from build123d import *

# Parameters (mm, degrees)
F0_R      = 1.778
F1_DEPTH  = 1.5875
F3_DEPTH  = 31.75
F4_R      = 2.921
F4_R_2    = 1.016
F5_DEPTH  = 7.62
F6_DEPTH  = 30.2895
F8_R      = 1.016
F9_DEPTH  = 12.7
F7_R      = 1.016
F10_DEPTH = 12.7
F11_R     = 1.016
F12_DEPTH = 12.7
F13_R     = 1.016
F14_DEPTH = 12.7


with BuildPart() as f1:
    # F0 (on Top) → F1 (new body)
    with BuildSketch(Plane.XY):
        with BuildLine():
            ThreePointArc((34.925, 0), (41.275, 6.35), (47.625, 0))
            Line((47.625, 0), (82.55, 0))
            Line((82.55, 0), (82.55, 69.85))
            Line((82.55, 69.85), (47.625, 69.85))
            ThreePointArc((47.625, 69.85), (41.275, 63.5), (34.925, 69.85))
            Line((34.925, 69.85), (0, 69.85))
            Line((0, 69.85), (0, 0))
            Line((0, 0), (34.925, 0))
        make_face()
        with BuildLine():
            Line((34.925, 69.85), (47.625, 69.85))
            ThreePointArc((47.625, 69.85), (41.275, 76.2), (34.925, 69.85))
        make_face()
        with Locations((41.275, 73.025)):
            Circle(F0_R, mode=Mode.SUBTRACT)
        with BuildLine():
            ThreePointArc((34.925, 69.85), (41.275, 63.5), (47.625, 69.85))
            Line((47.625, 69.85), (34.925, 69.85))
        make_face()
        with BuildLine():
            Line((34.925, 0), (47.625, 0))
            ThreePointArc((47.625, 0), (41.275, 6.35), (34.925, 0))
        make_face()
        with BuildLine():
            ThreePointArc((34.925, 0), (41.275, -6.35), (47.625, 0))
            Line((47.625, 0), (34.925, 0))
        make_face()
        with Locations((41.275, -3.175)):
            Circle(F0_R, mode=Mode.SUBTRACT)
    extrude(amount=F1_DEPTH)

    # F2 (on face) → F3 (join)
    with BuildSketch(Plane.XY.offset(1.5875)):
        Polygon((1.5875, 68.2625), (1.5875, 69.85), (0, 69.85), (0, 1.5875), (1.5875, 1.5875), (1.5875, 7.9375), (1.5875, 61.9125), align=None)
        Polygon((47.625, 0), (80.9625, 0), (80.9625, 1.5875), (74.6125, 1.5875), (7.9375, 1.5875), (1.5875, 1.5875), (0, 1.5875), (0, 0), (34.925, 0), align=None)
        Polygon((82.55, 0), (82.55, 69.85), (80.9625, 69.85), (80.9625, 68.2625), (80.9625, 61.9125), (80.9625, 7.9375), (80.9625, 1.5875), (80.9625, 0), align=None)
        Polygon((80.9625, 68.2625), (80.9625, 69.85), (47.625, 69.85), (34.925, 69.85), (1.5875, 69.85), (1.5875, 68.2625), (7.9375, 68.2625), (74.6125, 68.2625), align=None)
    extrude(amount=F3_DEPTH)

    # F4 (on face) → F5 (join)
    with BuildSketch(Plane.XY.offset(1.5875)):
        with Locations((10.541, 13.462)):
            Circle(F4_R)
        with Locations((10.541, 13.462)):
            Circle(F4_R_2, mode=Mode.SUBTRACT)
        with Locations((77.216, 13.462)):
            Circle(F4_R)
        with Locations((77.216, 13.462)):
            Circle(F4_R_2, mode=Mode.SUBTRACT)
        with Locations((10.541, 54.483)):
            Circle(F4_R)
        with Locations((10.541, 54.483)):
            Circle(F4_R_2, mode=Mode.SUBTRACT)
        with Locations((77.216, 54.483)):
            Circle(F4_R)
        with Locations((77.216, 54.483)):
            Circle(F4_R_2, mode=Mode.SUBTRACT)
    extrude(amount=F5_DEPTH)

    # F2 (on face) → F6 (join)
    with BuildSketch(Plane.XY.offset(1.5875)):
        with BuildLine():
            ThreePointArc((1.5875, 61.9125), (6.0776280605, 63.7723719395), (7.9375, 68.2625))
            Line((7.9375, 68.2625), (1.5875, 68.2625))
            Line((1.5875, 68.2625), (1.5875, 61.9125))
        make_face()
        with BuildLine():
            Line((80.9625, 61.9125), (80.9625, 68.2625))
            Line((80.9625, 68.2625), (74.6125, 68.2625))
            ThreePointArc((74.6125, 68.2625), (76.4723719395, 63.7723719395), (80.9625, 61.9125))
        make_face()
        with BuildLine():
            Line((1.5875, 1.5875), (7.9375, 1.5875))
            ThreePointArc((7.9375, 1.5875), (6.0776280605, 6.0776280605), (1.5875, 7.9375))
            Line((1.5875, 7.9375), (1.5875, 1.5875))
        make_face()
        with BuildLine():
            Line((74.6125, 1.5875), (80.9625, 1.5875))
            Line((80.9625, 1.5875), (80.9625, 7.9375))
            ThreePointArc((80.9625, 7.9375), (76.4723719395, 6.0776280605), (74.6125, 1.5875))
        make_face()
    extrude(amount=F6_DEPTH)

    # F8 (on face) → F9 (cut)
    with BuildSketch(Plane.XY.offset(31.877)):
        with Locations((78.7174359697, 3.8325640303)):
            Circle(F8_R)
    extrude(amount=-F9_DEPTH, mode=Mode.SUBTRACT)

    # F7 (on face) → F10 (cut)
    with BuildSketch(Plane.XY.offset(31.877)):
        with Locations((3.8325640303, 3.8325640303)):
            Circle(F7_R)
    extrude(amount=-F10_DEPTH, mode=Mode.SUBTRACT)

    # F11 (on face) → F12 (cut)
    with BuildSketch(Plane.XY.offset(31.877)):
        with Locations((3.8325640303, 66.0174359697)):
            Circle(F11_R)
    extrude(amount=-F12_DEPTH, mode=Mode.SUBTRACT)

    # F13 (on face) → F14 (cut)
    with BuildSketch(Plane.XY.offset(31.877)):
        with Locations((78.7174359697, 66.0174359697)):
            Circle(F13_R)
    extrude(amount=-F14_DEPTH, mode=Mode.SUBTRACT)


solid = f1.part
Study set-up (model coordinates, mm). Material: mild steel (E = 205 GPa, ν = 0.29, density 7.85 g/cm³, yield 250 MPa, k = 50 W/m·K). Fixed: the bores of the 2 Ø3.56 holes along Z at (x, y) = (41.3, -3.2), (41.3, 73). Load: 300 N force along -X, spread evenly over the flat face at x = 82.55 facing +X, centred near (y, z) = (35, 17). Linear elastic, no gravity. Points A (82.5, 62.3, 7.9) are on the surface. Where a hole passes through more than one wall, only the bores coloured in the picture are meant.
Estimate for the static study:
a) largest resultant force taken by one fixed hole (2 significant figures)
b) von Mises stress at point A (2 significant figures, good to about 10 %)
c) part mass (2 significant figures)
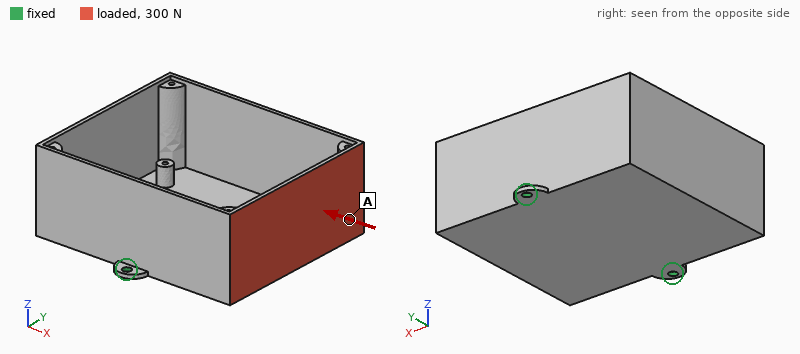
150 N
13 MPa
230 g
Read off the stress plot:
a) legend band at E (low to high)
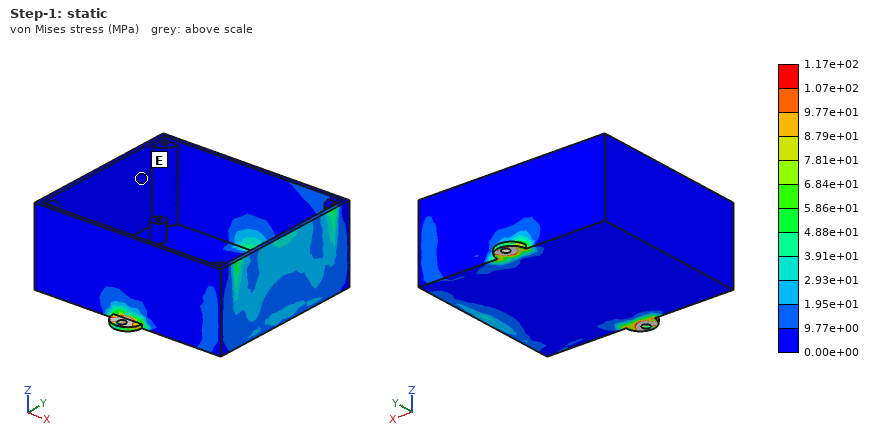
0.00e+00 to 9.77e+00 MPa
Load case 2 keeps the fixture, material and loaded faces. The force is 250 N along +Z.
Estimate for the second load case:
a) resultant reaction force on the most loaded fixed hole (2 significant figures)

130 N
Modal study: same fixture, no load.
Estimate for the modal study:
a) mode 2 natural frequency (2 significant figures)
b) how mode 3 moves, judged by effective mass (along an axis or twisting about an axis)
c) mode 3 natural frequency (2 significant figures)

730 Hz
along Z
1900 Hz
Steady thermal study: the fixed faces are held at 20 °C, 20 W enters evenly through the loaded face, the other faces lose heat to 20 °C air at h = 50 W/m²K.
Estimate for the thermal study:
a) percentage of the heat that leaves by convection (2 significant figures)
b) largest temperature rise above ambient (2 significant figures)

90 %
55 K
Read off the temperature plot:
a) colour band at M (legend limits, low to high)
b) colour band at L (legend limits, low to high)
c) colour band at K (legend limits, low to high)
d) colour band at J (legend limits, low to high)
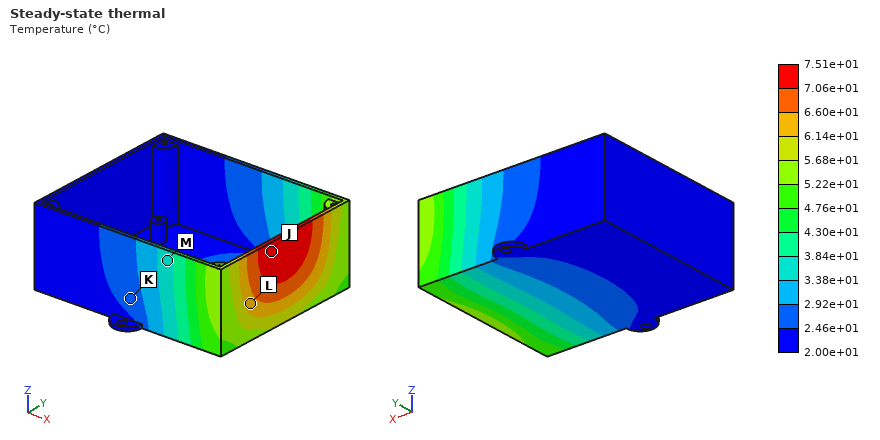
3.38e+01 to 3.84e+01 °C
6.14e+01 to 6.60e+01 °C
2.46e+01 to 2.92e+01 °C
7.06e+01 to 7.51e+01 °C
